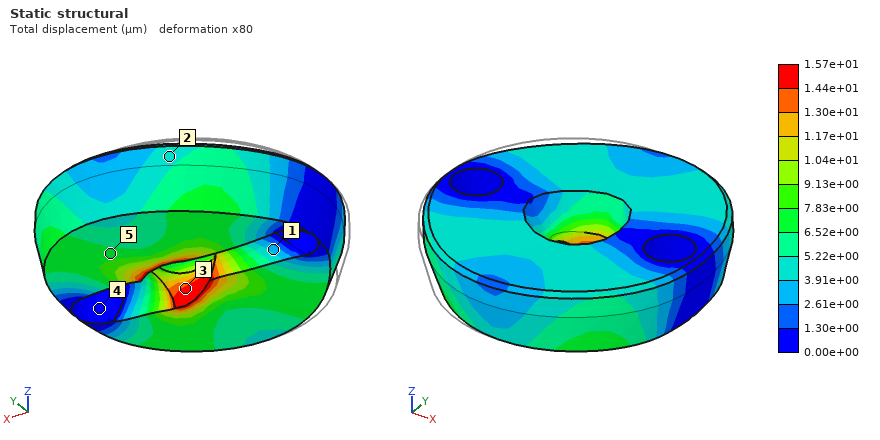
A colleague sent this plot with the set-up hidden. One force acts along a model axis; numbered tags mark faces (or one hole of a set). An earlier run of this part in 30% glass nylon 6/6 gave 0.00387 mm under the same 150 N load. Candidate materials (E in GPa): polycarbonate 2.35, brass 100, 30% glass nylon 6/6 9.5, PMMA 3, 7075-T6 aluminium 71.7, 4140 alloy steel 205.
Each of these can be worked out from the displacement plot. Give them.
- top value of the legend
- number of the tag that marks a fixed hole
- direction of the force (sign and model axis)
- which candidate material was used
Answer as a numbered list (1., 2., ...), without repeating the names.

1. 1.57e+01 µm
2. 4
3. +X
4. polycarbonate
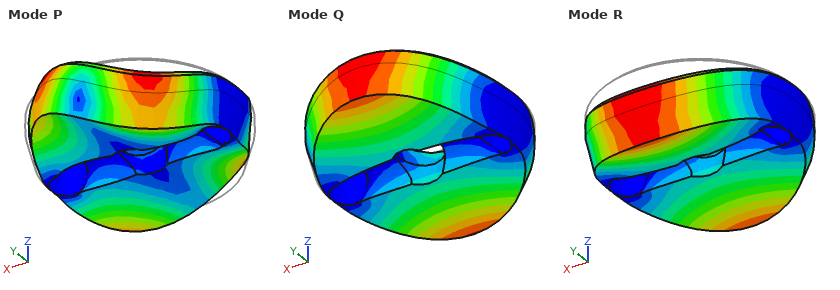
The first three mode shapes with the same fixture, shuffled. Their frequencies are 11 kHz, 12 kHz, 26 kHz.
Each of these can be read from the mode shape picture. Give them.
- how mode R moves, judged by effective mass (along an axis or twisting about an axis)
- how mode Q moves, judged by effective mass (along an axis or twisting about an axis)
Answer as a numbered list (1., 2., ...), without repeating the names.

1. along Z
2. twisting about X
